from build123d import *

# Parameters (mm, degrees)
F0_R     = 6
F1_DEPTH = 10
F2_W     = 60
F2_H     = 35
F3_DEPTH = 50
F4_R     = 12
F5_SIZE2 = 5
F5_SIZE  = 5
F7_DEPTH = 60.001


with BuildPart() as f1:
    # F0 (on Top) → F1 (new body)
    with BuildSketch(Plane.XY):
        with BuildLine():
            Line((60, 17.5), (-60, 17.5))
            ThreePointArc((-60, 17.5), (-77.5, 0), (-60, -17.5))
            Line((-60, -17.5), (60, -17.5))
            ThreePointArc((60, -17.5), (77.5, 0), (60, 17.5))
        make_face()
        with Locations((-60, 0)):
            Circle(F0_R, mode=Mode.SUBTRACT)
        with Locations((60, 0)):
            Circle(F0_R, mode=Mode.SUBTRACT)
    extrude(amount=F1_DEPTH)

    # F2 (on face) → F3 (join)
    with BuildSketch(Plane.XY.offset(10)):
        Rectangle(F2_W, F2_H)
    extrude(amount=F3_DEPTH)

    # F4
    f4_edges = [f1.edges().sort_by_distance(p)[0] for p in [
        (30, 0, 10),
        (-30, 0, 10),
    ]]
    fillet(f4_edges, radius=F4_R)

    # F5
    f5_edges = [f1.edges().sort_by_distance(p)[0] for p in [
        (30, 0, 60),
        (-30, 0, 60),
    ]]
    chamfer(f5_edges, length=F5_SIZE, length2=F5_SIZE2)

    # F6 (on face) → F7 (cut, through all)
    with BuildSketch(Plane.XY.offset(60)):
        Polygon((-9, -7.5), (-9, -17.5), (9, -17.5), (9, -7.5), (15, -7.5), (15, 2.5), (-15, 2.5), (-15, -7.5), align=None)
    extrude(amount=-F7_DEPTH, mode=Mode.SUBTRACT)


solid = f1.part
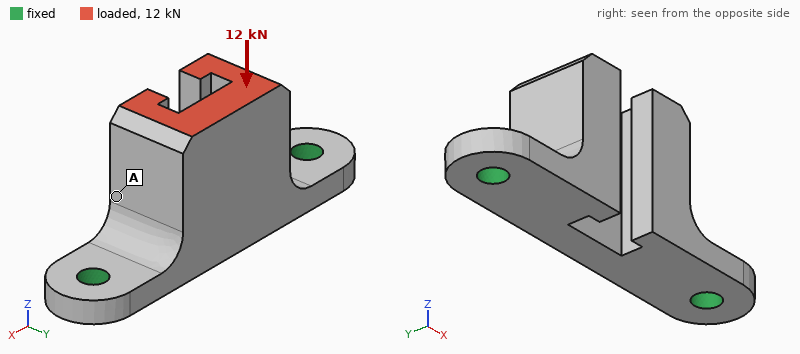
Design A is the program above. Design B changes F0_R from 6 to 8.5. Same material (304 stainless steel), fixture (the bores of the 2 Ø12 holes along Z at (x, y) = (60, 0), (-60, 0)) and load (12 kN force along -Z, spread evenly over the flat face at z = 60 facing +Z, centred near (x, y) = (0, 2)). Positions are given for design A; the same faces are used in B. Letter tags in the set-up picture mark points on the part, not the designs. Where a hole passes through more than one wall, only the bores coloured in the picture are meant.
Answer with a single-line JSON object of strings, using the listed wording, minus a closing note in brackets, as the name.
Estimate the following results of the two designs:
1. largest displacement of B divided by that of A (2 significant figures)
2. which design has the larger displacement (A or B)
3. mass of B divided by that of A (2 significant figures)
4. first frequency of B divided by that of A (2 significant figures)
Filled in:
{"largest displacement of B divided by that of A": "0.79", "which design has the larger displacement": "A", "mass of B divided by that of A": "0.98", "first frequency of B divided by that of A": "1.1"}
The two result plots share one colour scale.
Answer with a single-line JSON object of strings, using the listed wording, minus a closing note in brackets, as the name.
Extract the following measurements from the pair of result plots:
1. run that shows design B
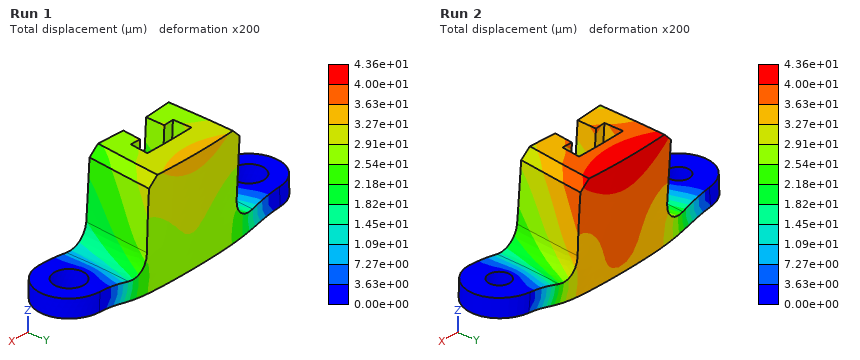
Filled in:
{"run that shows design B": "Run 1"}
